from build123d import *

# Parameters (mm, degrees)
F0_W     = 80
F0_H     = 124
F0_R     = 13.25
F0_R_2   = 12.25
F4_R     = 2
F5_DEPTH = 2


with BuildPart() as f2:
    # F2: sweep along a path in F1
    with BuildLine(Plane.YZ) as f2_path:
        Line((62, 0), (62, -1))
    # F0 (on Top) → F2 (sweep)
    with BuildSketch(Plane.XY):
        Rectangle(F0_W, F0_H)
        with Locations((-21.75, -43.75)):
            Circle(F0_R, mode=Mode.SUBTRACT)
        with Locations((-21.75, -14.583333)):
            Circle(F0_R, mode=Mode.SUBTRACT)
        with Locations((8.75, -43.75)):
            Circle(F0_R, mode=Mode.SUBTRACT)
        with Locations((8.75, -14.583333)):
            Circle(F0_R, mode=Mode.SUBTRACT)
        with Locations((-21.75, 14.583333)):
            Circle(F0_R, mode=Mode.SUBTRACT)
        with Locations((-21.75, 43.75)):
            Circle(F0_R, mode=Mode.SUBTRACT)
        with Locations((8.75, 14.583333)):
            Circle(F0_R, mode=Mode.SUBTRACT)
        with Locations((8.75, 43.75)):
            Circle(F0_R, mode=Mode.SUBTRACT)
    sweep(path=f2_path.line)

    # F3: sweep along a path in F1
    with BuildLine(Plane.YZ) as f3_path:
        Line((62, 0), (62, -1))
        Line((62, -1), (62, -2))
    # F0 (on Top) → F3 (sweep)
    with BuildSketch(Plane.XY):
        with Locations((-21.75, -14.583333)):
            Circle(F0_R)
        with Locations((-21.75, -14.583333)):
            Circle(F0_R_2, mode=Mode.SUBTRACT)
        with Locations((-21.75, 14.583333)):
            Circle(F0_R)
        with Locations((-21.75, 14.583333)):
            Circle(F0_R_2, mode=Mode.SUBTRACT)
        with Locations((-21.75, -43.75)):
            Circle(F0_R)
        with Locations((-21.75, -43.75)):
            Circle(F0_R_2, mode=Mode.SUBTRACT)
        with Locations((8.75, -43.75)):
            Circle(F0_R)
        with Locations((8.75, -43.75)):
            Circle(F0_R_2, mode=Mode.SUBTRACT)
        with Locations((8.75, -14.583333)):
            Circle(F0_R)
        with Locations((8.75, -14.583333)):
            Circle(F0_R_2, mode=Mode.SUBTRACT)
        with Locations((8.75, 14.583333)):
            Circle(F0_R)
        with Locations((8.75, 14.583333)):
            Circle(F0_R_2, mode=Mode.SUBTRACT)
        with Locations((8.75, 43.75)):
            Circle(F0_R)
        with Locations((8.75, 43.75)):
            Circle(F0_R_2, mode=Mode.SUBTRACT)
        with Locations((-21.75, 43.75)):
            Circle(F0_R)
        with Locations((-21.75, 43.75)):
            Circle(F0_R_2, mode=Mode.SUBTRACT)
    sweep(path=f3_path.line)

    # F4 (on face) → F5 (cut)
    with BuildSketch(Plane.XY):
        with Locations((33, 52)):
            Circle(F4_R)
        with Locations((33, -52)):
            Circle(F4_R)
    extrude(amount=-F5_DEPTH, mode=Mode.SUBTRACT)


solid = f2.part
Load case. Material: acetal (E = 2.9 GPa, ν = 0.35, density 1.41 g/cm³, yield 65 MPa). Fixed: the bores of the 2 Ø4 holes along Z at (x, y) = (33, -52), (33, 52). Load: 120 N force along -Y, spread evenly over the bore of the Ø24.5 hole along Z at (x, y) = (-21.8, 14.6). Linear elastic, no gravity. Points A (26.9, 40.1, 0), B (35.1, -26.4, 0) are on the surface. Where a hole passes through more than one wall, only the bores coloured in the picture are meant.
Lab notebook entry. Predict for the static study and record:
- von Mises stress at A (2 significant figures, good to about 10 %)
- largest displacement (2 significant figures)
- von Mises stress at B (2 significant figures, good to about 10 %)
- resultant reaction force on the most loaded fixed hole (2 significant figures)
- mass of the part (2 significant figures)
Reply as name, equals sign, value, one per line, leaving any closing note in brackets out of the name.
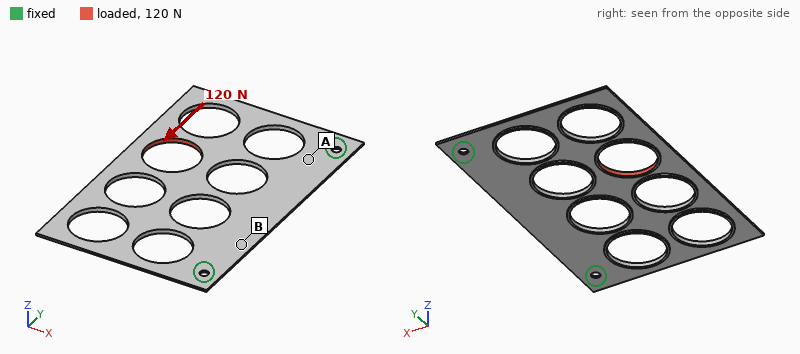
von Mises stress at A = 4.3 MPa
largest displacement = 1.6 mm
von Mises stress at B = 1.9 MPa
resultant reaction force on the most loaded fixed hole = 86 N
mass of the part = 9.5 g
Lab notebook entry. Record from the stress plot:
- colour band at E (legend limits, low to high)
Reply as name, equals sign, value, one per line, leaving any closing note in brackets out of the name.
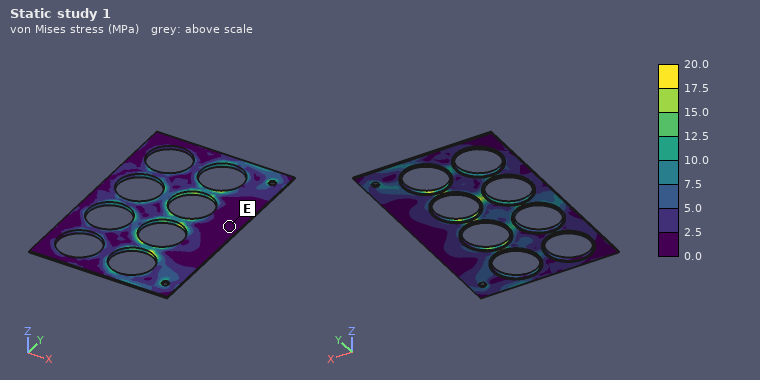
colour band at E = 0.0 to 2.5 MPa
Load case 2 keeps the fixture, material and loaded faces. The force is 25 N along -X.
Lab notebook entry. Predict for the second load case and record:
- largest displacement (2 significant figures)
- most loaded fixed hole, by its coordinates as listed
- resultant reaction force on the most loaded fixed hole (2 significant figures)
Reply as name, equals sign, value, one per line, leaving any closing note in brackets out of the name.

largest displacement = 1.7 mm
most loaded fixed hole, by its coordinates as listed = (33, 52)
resultant reaction force on the most loaded fixed hole = 17 N
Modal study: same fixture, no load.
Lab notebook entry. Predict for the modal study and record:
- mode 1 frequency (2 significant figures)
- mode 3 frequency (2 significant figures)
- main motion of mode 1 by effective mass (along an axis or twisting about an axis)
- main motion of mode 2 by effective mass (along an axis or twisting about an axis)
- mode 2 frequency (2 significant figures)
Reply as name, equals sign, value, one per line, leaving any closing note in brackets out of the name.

mode 1 frequency = 38 Hz
mode 3 frequency = 130 Hz
main motion of mode 1 by effective mass = along Z
main motion of mode 2 by effective mass = twisting about X
mode 2 frequency = 78 Hz
